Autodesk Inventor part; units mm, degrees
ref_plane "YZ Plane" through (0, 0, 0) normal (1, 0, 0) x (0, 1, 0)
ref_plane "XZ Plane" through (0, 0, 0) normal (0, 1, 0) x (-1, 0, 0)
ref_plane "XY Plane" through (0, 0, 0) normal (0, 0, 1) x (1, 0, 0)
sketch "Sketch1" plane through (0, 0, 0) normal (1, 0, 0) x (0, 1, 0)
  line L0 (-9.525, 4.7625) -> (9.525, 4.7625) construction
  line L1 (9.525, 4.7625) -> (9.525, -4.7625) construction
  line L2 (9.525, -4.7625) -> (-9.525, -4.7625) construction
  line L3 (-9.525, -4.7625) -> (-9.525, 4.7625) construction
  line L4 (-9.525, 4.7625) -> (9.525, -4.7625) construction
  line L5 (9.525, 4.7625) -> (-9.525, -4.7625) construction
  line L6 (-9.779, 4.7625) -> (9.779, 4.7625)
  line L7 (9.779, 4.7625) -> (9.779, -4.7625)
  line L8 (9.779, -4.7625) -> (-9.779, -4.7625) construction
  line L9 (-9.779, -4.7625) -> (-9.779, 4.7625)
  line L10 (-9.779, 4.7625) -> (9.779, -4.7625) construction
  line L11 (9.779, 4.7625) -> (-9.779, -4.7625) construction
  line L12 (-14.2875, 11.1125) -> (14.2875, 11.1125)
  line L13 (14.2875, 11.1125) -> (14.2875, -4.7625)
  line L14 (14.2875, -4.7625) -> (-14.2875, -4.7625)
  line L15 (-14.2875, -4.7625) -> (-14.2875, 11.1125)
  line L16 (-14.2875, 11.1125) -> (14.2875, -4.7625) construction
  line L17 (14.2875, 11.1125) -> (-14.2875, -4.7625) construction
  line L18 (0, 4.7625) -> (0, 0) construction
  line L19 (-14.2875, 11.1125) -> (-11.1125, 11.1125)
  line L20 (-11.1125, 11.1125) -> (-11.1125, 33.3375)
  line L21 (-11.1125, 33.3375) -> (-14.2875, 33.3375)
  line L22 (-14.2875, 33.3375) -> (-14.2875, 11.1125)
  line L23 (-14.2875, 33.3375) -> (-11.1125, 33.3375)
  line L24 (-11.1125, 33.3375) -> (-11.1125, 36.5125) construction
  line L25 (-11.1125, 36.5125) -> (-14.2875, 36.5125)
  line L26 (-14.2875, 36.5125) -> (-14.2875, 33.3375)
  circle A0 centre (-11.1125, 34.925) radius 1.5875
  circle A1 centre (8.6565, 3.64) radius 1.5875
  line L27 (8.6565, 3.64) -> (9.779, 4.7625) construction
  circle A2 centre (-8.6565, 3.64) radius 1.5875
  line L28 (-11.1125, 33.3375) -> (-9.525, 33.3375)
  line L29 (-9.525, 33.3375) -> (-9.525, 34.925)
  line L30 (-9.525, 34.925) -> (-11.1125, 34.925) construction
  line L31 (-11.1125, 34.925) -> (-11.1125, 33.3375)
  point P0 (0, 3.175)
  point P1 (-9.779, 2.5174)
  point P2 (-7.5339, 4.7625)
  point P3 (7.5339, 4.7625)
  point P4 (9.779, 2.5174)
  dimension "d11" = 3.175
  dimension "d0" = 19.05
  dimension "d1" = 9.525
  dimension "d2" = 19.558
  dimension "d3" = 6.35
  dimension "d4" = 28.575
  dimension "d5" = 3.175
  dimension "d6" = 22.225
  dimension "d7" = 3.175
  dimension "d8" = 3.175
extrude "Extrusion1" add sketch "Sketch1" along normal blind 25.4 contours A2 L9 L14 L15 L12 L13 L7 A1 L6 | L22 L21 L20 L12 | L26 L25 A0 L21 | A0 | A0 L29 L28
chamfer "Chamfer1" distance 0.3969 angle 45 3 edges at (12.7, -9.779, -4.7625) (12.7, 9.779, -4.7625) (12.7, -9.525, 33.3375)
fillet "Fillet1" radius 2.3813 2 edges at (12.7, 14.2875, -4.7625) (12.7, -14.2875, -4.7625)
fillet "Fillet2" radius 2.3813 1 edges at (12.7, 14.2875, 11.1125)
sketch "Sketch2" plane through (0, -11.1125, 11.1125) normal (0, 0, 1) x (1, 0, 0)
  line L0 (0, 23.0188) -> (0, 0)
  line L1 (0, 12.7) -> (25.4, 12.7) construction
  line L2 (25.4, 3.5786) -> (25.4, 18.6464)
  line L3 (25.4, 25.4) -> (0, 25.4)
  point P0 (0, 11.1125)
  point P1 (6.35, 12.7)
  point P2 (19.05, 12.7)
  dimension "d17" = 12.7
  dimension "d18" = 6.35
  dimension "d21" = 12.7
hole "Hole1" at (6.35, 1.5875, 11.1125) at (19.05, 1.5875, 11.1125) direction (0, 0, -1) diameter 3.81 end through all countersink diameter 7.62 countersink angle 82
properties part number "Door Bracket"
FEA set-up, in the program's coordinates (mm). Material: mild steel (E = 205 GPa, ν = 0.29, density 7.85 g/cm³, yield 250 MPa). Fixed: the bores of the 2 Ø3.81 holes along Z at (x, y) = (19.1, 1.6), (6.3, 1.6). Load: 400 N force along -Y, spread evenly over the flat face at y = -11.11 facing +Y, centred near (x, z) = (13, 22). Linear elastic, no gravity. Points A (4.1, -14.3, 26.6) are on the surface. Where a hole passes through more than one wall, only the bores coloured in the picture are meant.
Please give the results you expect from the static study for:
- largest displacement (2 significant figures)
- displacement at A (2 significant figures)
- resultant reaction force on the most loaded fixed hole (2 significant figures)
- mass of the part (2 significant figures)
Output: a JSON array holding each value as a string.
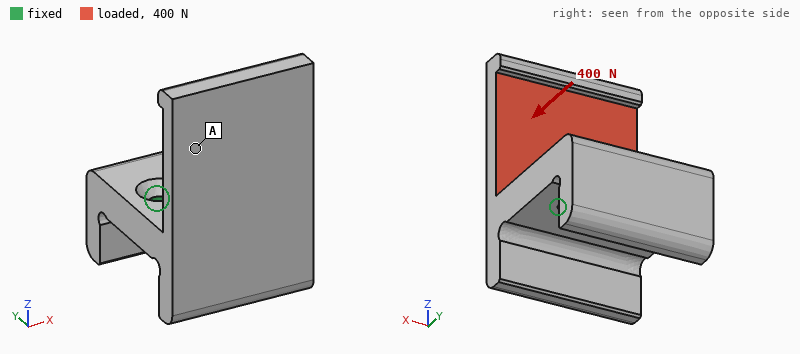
["84 µm", "49 µm", "200 N", "67 g"]
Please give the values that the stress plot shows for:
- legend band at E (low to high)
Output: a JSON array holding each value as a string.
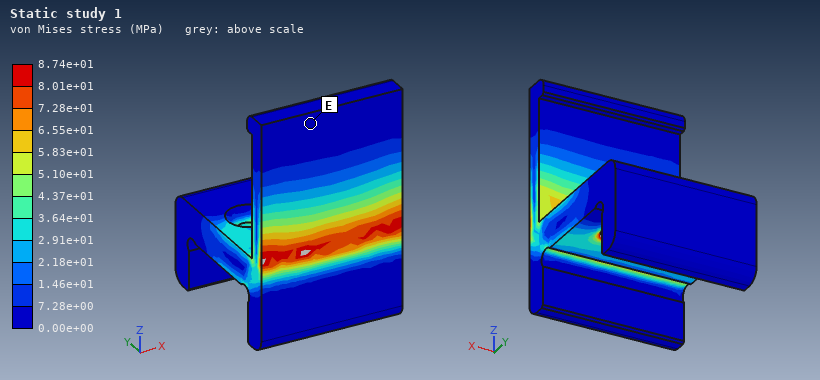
["0.00e+00 to 7.28e+00 MPa"]
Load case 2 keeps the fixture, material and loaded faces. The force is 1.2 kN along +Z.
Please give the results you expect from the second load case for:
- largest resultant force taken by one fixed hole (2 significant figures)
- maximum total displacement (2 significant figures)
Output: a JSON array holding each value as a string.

["600 N", "21 µm"]
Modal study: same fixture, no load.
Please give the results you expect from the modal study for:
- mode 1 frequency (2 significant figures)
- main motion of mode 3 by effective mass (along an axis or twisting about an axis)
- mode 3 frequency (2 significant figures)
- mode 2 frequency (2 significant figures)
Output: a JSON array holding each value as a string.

["2800 Hz", "along Z", "7700 Hz", "6400 Hz"]
